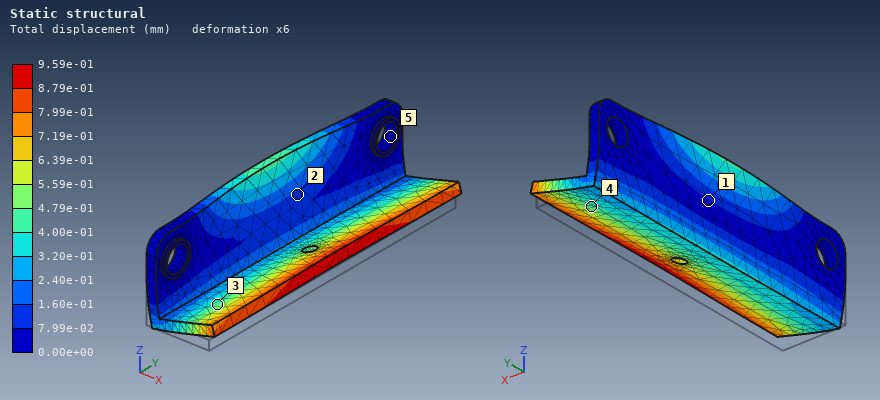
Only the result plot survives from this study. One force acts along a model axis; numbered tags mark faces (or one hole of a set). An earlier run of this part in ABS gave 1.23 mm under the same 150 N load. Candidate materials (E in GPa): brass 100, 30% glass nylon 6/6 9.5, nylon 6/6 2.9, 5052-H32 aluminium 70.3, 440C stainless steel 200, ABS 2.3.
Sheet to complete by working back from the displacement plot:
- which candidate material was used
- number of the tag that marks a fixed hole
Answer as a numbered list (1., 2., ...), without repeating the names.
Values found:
1. nylon 6/6
2. 5
